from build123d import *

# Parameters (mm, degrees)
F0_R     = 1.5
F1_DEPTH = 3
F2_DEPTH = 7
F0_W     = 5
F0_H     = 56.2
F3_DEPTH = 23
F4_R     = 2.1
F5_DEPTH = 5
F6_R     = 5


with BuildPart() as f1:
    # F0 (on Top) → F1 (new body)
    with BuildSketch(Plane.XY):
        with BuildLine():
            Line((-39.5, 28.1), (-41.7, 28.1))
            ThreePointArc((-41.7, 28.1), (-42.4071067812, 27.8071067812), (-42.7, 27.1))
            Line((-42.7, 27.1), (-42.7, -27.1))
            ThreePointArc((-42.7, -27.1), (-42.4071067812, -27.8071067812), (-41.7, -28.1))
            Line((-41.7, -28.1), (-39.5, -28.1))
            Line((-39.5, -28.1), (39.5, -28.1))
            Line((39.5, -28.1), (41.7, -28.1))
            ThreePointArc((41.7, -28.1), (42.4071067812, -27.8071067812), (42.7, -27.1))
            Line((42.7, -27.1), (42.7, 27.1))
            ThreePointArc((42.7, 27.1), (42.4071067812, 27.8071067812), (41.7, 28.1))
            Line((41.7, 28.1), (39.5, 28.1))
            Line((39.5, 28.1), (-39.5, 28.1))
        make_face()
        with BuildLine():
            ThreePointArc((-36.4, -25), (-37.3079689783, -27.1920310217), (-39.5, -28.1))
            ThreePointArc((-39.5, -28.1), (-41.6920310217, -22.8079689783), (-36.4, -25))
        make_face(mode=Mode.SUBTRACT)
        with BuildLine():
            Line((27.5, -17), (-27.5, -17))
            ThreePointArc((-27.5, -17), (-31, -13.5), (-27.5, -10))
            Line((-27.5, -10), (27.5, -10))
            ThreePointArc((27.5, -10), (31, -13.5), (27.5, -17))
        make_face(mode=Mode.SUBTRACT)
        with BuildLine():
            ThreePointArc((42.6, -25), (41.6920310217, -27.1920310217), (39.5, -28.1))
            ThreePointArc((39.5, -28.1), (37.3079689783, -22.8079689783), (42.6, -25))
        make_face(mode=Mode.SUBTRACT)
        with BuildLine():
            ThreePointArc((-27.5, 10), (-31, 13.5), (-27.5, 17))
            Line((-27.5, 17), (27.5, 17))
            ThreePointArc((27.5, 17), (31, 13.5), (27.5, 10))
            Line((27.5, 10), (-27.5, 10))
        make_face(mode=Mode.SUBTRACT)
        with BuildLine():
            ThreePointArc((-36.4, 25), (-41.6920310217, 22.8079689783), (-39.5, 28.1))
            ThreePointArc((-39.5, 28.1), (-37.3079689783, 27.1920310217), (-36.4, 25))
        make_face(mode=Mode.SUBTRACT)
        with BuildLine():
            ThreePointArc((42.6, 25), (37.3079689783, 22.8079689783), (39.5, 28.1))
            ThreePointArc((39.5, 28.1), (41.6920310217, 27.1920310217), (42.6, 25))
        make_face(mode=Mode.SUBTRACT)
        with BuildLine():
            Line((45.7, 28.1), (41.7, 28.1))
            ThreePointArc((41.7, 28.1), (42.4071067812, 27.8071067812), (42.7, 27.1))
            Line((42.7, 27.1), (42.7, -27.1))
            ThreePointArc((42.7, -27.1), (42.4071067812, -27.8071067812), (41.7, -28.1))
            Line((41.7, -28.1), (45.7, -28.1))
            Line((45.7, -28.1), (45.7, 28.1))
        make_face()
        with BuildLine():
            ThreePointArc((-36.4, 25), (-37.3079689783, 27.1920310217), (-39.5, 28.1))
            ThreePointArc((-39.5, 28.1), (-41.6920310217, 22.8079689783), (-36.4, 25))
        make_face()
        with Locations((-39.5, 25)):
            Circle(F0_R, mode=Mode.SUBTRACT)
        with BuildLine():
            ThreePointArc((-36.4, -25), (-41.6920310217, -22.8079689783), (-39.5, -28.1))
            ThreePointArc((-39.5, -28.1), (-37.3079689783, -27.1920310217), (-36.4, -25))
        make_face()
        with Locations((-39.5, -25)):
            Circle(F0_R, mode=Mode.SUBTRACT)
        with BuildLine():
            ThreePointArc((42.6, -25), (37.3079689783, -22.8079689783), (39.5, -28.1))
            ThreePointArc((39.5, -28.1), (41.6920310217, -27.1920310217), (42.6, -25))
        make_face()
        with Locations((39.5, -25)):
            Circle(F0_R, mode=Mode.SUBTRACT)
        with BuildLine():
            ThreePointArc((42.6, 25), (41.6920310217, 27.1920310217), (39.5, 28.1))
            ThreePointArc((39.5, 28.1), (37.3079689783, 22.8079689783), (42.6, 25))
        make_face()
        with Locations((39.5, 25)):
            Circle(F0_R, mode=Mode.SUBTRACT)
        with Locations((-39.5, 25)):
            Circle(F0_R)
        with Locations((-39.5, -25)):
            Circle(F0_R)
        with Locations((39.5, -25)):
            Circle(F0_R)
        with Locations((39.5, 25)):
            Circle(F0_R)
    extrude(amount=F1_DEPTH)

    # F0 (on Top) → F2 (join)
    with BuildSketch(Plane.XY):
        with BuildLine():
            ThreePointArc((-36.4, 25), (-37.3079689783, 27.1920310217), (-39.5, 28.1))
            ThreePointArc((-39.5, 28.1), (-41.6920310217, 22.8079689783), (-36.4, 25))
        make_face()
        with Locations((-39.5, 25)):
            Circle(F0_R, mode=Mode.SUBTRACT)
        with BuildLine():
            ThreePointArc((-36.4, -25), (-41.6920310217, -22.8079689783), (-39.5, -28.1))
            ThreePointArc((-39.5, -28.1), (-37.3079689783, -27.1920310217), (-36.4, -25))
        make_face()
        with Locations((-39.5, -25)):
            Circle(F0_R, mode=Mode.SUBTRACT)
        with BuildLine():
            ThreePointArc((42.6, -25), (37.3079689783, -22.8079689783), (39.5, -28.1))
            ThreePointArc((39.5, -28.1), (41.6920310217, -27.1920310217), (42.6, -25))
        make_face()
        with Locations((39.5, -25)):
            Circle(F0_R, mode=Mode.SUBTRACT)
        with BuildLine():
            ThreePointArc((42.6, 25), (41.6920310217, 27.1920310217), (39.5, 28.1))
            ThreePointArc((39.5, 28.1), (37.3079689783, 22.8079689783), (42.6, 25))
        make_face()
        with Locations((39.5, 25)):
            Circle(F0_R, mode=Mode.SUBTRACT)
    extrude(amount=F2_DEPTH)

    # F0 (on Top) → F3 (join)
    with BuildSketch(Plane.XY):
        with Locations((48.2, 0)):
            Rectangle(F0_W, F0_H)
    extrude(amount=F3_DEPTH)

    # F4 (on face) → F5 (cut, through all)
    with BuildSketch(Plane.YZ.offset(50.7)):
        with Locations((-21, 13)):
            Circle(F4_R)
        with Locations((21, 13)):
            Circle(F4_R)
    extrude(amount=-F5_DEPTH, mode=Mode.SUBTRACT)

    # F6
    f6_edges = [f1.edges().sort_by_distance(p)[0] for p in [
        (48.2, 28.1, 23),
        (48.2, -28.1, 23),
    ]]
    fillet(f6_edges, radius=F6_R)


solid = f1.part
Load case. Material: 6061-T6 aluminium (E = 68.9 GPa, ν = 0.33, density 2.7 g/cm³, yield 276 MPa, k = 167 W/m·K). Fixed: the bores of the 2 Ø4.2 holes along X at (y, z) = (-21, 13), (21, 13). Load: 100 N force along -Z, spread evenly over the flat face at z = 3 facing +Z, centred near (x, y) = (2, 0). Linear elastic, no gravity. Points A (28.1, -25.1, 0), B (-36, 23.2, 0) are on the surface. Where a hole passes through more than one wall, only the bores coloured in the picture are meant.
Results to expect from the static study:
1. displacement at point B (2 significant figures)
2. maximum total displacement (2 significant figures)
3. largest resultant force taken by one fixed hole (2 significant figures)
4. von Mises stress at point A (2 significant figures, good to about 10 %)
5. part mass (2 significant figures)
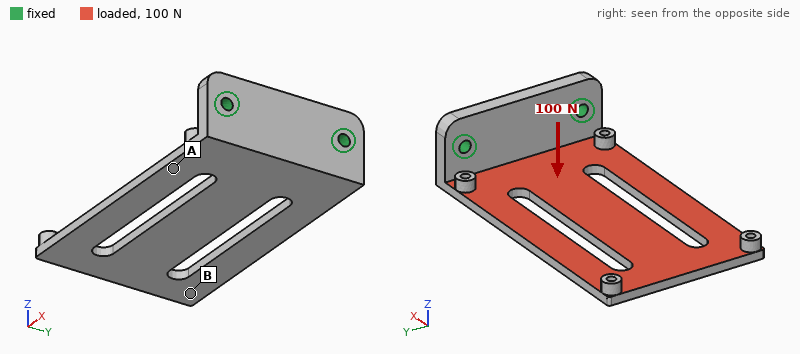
1.1 mm
1.3 mm
52 N
43 MPa
51 g
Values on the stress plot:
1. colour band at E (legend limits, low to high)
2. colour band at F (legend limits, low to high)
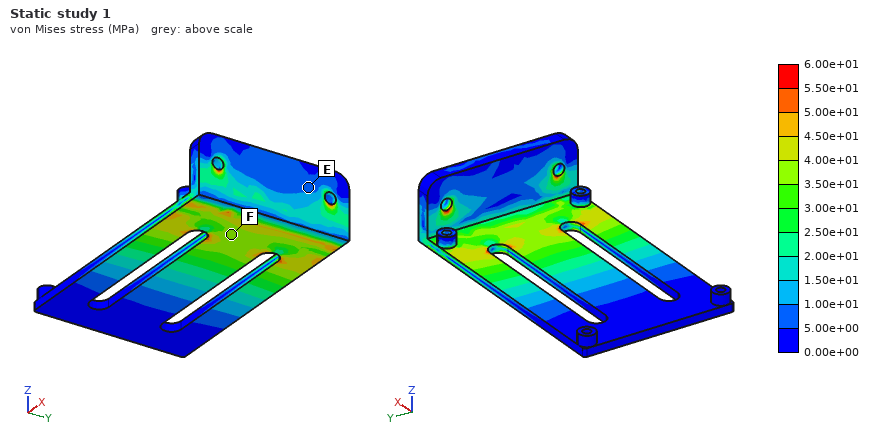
5.00e+00 to 1.00e+01 MPa
3.50e+01 to 4.00e+01 MPa
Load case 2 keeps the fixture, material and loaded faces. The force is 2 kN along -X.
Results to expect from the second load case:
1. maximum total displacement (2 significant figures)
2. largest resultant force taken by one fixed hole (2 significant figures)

0.73 mm
1.0 kN
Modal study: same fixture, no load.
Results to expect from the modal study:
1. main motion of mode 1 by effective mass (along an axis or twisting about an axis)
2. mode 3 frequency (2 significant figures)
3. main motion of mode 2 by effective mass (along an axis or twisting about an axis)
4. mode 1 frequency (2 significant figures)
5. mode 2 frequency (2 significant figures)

along Z
1800 Hz
twisting about X
290 Hz
930 Hz
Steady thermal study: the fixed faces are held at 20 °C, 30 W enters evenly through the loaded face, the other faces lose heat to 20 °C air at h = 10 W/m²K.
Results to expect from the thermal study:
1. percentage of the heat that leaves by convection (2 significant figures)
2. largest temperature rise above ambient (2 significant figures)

9.4 %
61 K
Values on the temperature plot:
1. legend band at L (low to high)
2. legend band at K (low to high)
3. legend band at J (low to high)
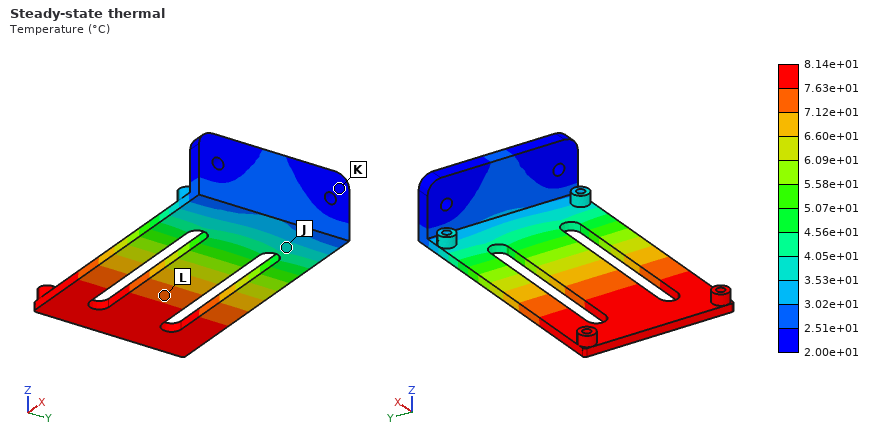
7.12e+01 to 7.63e+01 °C
2.00e+01 to 2.51e+01 °C
3.53e+01 to 4.05e+01 °C
